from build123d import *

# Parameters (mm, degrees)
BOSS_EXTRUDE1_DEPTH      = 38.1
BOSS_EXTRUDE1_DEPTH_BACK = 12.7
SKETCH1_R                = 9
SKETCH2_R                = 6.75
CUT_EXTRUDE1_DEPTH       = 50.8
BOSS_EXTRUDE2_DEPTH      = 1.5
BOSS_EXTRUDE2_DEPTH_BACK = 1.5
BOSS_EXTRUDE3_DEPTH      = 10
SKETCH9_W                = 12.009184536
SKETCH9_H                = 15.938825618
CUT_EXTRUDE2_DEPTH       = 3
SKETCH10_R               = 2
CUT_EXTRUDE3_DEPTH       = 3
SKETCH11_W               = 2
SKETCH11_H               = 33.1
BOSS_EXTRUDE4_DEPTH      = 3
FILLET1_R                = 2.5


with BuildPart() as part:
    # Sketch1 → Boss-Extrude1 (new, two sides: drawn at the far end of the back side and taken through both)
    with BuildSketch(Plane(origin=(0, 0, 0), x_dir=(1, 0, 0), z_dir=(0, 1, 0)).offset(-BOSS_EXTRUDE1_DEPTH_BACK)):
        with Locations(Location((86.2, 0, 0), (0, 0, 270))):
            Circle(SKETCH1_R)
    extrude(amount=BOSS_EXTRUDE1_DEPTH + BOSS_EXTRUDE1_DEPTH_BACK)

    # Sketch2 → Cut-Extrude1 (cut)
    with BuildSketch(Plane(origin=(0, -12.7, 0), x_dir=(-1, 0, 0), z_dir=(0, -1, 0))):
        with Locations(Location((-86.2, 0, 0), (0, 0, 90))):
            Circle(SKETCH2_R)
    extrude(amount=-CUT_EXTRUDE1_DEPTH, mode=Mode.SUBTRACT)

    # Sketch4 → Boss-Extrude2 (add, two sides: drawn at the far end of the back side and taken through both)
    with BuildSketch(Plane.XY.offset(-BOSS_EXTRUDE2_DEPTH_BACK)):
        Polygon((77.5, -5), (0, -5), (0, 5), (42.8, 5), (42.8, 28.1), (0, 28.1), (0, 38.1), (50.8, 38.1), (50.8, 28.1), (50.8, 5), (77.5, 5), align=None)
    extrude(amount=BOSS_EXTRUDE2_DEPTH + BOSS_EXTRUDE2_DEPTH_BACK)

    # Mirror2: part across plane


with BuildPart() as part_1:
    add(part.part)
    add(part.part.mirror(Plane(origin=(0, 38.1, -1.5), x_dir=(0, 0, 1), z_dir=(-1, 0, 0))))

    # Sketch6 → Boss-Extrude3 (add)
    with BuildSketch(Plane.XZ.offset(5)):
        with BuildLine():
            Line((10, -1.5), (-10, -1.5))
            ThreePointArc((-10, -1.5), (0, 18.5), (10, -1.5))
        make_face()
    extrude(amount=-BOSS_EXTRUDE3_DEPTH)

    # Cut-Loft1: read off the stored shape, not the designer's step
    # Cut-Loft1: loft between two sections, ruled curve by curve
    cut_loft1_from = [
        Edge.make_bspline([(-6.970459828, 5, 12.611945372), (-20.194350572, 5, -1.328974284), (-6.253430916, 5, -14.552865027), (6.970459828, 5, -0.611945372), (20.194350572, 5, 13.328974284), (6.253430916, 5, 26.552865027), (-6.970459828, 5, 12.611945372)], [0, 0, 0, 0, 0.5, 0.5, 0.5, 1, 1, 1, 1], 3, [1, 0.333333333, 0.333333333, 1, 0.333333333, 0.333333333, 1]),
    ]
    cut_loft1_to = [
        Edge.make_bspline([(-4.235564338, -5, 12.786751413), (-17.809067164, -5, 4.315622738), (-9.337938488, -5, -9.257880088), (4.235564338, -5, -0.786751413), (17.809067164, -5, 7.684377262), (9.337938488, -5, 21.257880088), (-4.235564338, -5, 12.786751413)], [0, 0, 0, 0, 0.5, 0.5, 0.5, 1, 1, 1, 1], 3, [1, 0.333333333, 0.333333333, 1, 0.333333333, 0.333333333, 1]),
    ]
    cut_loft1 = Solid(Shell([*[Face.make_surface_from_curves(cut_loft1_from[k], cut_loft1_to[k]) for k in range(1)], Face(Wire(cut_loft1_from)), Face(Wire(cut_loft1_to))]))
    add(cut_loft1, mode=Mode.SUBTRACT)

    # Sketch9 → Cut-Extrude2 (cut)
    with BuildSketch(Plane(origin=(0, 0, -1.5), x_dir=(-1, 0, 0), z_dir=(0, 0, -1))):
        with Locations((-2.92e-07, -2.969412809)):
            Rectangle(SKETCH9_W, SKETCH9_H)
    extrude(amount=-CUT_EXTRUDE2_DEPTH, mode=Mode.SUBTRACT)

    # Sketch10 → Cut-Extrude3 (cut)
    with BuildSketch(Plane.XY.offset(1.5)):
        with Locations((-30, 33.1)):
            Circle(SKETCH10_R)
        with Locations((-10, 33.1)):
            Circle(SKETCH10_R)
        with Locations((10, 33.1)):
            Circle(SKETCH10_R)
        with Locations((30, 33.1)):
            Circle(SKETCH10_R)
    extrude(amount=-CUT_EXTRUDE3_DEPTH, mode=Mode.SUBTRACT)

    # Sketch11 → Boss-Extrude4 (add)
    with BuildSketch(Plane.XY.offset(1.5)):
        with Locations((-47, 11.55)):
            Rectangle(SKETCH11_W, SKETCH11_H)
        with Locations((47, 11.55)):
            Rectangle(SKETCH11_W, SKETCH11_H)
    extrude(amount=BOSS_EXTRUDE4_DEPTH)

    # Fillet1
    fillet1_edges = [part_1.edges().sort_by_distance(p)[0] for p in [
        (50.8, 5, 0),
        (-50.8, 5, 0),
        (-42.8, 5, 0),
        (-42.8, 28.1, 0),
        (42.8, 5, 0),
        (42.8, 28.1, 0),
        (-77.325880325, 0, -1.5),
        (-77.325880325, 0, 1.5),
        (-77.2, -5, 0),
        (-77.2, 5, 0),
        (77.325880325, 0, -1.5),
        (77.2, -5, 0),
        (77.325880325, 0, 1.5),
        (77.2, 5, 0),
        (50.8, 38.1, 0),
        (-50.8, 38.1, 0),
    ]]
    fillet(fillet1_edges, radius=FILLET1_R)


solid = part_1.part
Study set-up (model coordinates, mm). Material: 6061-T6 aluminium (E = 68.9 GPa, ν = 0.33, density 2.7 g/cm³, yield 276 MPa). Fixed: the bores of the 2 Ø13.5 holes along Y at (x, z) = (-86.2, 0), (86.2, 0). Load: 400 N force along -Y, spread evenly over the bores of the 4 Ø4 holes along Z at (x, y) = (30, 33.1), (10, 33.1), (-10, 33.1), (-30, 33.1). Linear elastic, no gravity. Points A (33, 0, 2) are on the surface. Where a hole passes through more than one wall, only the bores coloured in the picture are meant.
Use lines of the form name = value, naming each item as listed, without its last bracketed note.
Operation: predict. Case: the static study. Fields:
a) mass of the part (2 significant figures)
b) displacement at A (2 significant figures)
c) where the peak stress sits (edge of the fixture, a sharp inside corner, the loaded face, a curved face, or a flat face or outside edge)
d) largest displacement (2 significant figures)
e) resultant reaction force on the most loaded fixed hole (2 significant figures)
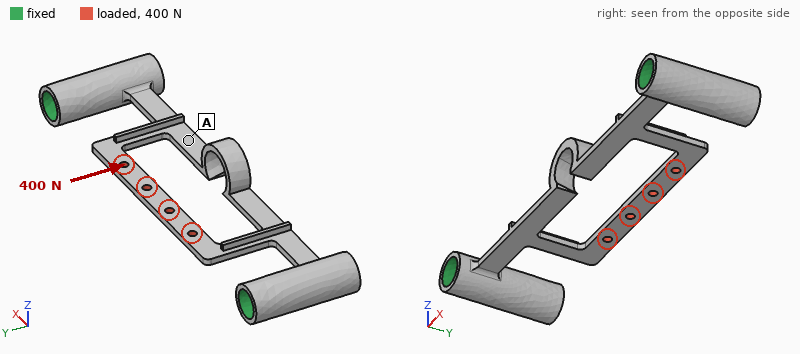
mass of the part = 58 g
displacement at A = 0.050 mm
where the peak stress sits = a curved face
largest displacement = 0.14 mm
resultant reaction force on the most loaded fixed hole = 260 N
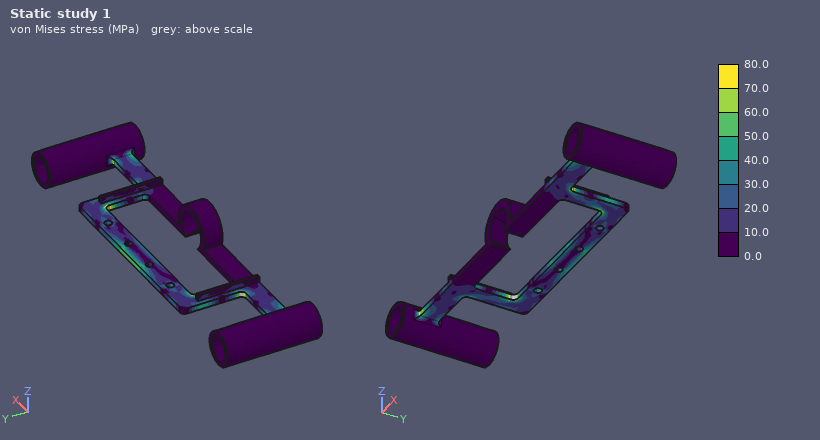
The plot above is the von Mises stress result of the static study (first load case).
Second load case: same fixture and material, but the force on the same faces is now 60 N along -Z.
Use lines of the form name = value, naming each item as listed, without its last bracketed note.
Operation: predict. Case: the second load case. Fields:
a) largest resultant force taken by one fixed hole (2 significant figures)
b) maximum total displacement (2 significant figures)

largest resultant force taken by one fixed hole = 38 N
maximum total displacement = 1.1 mm
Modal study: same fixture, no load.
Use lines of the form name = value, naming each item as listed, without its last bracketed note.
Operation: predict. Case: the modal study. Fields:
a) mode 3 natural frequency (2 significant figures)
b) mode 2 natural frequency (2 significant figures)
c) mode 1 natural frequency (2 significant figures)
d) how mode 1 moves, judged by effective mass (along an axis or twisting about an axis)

mode 3 natural frequency = 1100 Hz
mode 2 natural frequency = 730 Hz
mode 1 natural frequency = 410 Hz
how mode 1 moves, judged by effective mass = along Z
